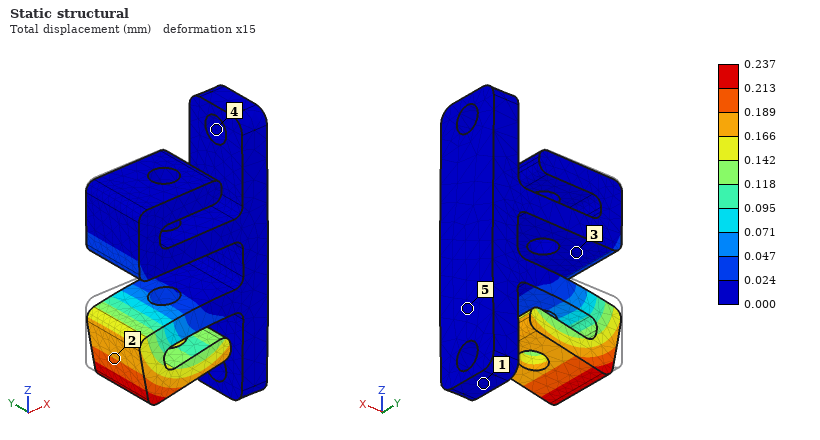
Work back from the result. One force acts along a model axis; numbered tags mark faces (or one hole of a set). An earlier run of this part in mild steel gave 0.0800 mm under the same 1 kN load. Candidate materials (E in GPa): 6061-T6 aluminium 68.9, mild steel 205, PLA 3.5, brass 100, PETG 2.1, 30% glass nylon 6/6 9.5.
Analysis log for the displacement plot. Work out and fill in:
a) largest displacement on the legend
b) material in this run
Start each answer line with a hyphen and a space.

- 0.237 mm
- 6061-T6 aluminium
